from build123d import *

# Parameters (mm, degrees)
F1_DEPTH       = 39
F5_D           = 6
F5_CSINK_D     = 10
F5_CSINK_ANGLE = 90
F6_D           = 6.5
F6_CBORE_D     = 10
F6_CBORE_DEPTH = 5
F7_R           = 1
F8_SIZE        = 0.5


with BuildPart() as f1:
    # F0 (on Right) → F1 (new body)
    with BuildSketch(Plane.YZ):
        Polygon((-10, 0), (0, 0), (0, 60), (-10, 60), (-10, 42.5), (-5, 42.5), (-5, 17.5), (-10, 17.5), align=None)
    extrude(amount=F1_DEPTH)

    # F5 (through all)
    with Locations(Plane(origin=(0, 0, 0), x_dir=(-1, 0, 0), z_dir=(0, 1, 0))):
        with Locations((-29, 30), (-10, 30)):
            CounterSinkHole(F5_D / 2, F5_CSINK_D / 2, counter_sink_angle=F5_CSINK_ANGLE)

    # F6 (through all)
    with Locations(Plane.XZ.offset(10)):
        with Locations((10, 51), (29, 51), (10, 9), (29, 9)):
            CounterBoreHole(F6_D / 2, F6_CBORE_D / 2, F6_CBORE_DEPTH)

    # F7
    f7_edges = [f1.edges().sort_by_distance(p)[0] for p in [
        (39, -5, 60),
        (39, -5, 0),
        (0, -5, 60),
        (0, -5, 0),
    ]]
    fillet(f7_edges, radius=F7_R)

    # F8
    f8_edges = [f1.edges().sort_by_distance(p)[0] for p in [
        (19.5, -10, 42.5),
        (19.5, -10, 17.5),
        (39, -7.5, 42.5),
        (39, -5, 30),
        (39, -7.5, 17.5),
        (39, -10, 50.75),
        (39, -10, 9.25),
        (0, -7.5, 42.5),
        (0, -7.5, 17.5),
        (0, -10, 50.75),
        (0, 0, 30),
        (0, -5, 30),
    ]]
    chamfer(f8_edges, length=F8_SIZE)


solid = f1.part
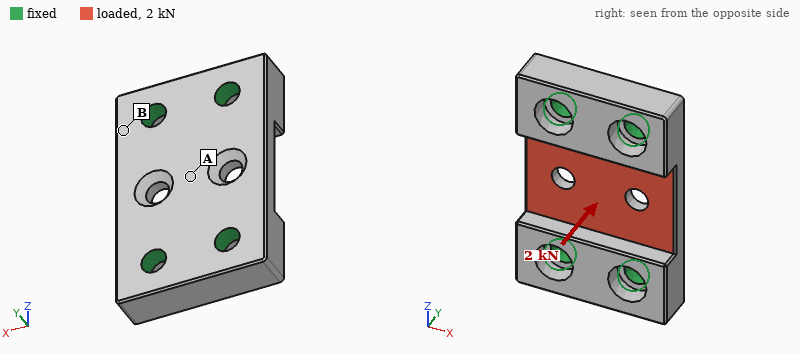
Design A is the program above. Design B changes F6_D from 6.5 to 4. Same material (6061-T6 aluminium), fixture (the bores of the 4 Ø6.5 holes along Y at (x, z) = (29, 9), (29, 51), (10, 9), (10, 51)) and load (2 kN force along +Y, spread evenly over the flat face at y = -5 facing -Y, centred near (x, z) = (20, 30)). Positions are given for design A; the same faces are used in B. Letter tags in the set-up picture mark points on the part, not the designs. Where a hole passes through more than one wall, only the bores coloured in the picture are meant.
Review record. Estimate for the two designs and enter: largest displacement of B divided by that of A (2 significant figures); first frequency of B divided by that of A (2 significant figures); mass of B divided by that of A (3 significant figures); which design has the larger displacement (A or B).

1.4
0.79
1.03
B
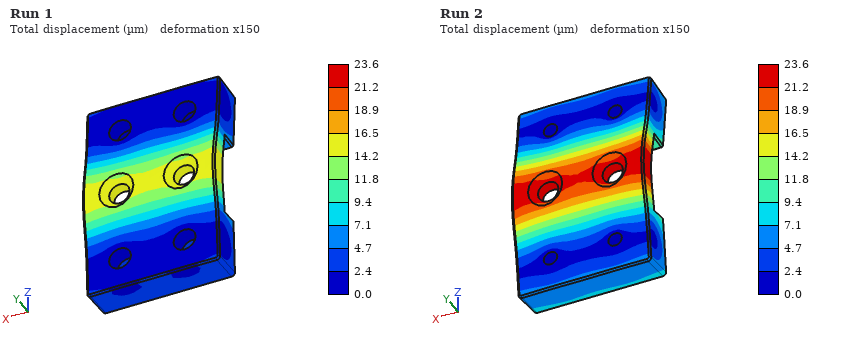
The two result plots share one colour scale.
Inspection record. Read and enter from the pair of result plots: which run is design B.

Run 2
